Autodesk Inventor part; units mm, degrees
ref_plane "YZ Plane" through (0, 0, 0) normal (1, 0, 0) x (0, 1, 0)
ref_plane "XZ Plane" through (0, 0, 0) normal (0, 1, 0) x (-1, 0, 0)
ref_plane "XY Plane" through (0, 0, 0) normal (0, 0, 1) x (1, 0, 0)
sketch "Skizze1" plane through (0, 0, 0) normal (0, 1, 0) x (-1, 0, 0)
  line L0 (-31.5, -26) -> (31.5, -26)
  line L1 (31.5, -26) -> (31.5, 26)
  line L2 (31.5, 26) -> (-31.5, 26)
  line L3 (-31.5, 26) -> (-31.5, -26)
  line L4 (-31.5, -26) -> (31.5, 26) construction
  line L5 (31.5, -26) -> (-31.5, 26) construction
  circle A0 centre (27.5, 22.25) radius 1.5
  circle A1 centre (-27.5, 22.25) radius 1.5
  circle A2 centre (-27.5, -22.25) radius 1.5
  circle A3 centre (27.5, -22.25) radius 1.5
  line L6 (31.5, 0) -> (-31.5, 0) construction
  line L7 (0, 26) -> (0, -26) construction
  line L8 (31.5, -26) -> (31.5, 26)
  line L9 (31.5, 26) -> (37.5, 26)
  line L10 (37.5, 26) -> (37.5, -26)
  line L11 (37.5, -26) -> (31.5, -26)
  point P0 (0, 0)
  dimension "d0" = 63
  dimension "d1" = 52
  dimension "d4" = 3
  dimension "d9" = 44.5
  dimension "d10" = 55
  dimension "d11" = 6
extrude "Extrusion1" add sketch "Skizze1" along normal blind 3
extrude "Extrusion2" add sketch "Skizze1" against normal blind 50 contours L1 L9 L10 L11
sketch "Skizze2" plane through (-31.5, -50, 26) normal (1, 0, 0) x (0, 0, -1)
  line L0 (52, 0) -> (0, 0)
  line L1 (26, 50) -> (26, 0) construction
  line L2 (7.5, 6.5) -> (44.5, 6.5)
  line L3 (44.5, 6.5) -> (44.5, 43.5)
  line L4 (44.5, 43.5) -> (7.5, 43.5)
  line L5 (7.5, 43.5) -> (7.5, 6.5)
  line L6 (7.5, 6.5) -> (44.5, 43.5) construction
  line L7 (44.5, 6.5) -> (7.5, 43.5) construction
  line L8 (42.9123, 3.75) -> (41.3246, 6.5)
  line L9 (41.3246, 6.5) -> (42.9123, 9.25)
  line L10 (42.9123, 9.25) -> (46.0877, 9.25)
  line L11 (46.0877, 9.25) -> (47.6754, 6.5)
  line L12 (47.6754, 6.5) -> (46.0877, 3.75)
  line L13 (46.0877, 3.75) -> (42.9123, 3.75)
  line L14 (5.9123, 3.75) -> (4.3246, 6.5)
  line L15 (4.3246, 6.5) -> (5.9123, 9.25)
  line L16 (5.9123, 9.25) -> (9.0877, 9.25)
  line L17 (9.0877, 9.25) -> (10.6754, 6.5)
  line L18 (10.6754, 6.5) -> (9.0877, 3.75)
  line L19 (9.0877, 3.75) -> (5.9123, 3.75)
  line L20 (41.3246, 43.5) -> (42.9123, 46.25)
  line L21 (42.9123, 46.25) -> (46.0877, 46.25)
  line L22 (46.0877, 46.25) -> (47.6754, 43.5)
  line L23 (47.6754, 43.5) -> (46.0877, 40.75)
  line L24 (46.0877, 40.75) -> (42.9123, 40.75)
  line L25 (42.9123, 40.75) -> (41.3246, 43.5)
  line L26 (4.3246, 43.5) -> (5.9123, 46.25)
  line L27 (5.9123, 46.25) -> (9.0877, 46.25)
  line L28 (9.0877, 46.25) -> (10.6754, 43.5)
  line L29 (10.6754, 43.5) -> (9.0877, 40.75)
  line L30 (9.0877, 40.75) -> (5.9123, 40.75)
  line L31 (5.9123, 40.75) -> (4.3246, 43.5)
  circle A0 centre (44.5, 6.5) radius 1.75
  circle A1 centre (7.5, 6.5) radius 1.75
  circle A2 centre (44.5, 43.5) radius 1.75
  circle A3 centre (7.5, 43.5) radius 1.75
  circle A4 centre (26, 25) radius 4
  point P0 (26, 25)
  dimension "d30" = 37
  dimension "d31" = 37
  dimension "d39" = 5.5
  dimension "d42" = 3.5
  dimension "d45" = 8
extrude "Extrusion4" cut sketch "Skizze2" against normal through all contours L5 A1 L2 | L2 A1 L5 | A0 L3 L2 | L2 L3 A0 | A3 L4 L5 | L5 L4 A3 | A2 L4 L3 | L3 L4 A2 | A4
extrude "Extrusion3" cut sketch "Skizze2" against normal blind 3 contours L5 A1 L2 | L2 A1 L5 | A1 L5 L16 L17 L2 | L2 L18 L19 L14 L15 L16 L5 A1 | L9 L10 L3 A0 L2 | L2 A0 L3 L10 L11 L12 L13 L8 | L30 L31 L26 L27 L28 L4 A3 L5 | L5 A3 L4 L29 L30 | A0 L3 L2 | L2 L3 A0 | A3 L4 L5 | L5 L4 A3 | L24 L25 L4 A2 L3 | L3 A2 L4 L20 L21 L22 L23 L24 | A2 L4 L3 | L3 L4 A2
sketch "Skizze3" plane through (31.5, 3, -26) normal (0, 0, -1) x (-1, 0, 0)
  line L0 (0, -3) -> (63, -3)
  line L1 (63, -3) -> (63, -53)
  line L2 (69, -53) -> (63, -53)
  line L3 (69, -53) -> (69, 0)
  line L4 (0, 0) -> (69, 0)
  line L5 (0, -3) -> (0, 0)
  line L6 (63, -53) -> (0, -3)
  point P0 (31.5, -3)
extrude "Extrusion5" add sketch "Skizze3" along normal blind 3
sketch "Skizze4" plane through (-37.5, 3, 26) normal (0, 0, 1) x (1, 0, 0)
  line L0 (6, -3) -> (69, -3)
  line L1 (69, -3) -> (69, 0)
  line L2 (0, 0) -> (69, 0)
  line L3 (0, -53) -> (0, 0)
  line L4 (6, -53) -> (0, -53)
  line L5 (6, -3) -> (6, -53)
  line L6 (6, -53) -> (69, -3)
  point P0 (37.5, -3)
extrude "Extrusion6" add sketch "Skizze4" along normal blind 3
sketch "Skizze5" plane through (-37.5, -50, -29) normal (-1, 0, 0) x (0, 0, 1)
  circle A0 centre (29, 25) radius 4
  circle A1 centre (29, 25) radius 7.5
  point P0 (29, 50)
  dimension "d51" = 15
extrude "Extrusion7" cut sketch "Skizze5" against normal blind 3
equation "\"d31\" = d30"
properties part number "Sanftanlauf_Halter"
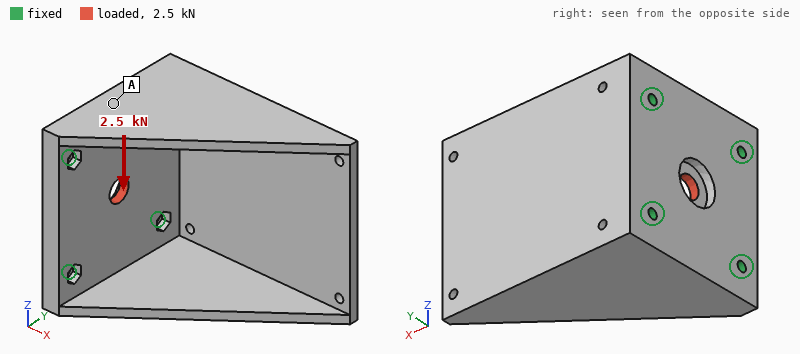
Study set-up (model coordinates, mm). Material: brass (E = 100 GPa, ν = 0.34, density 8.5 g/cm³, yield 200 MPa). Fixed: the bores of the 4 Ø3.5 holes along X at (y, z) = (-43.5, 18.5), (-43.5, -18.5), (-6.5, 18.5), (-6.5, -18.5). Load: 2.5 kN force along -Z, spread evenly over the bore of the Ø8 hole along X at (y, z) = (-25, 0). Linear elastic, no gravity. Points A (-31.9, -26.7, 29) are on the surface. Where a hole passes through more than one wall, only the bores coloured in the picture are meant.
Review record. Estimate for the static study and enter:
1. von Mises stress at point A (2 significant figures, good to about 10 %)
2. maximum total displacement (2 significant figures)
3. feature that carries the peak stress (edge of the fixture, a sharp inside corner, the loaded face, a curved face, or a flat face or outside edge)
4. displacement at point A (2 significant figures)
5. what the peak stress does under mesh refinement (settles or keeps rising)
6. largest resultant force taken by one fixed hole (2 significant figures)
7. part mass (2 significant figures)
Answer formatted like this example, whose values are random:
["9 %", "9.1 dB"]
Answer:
["5.0 MPa", "4.8 µm", "edge of the fixture", "2.4 µm", "keeps rising", "670 N", "320 g"]
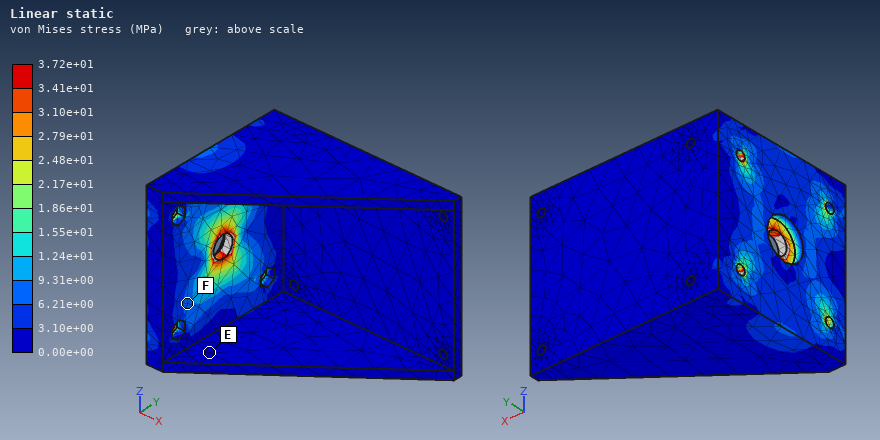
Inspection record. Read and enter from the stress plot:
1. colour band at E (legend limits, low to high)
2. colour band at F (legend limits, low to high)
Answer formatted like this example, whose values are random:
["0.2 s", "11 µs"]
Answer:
["0.00e+00 to 3.10e+00 MPa", "6.21e+00 to 9.31e+00 MPa"]
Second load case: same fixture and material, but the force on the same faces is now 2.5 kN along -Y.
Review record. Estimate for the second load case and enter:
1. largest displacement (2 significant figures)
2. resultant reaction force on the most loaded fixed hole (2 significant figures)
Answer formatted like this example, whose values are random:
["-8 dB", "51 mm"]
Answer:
["5.0 µm", "690 N"]
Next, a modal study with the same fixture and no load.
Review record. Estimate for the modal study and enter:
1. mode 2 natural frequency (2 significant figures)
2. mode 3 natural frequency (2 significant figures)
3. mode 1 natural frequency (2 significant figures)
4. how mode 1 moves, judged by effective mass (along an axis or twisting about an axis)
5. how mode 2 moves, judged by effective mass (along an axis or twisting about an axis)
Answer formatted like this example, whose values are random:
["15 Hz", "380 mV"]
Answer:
["2300 Hz", "3300 Hz", "1800 Hz", "along Y", "along Z"]
